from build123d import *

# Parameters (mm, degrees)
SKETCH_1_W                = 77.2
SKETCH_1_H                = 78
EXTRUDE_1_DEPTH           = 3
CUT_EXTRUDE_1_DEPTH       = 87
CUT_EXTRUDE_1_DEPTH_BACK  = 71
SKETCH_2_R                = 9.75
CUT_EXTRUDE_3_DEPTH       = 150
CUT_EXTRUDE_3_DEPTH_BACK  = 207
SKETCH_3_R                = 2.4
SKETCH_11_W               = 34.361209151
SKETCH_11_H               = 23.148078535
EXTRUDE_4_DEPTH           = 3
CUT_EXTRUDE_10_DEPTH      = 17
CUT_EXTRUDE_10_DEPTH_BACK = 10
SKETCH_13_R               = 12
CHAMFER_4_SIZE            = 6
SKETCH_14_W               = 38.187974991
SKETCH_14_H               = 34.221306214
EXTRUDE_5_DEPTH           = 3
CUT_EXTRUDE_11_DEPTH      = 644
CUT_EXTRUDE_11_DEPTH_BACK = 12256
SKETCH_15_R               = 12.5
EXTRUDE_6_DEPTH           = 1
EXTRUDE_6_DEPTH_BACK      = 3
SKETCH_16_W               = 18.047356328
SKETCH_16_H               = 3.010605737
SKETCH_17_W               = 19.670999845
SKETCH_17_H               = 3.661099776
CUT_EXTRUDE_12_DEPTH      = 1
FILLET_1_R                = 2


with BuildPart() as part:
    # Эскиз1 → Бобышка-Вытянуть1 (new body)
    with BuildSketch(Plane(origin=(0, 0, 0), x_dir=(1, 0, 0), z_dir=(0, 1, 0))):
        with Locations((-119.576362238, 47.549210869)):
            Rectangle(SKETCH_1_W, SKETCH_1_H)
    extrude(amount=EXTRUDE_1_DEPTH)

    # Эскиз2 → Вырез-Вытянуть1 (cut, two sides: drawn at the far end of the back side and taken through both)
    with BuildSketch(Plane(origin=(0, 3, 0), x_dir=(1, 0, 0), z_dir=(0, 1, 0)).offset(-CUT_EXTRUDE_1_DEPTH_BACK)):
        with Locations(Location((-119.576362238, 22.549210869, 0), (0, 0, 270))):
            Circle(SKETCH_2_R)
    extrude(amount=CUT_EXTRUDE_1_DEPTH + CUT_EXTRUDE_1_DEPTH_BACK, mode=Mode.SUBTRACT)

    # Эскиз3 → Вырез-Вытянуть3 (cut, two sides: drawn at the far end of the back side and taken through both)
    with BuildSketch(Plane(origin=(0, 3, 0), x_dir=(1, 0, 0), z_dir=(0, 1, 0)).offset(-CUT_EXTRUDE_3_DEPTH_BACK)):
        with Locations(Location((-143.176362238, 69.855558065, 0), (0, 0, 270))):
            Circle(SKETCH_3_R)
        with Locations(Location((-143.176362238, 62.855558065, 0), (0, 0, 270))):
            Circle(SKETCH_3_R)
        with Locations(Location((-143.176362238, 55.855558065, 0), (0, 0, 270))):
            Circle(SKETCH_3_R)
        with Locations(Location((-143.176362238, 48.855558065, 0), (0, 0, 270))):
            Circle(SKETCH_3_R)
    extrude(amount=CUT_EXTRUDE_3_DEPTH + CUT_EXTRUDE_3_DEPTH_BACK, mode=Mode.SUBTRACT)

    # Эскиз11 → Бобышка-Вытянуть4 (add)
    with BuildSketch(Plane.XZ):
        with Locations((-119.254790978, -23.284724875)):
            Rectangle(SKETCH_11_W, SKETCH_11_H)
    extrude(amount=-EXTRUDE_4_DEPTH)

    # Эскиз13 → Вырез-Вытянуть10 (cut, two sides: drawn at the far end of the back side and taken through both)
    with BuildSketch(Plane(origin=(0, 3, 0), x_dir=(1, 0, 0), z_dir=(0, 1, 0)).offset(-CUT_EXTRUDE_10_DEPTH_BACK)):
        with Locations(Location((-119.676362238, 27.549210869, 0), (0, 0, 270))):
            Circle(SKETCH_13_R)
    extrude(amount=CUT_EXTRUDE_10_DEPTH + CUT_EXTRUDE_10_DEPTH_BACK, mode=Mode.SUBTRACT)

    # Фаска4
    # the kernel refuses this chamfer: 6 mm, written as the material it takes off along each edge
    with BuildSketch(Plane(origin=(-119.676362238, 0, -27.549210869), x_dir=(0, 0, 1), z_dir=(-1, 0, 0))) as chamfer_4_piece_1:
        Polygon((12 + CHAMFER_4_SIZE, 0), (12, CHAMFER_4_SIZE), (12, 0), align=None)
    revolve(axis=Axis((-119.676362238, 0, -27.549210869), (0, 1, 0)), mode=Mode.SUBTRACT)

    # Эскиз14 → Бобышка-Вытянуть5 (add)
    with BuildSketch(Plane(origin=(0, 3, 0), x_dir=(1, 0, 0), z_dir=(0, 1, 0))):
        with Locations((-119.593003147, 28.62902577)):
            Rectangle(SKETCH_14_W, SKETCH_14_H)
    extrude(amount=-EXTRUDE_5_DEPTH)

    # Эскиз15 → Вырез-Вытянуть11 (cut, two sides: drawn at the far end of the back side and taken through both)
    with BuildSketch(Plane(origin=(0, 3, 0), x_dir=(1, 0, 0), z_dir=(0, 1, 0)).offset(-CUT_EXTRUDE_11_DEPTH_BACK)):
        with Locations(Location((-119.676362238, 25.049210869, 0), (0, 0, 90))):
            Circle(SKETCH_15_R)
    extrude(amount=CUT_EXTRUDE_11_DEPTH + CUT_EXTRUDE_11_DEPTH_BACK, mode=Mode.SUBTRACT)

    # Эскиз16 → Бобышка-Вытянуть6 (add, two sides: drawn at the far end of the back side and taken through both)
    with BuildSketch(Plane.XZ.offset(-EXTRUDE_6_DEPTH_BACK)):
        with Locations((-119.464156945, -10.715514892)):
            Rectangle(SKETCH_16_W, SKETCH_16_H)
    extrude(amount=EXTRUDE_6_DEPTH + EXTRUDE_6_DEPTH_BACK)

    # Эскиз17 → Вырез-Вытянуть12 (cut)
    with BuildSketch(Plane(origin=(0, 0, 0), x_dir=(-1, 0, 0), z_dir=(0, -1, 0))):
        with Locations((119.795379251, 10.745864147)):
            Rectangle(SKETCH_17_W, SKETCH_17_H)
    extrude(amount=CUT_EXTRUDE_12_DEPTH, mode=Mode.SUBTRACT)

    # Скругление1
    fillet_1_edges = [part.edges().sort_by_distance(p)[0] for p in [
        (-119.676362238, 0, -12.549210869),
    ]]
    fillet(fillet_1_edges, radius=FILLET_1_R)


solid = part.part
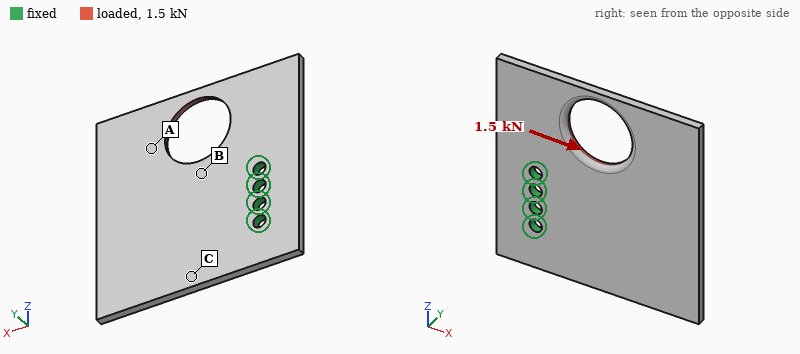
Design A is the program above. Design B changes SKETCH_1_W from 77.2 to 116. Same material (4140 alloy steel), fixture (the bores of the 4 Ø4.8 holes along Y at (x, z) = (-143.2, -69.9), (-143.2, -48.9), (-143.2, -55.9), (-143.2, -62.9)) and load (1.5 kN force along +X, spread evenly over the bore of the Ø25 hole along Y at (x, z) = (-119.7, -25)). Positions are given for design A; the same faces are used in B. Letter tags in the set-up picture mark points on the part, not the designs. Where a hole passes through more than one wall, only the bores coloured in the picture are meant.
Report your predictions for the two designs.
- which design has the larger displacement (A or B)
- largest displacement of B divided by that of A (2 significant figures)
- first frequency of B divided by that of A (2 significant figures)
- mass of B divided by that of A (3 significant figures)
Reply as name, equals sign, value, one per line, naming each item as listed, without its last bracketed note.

which design has the larger displacement = B
largest displacement of B divided by that of A = 1.2
first frequency of B divided by that of A = 0.59
mass of B divided by that of A = 1.56
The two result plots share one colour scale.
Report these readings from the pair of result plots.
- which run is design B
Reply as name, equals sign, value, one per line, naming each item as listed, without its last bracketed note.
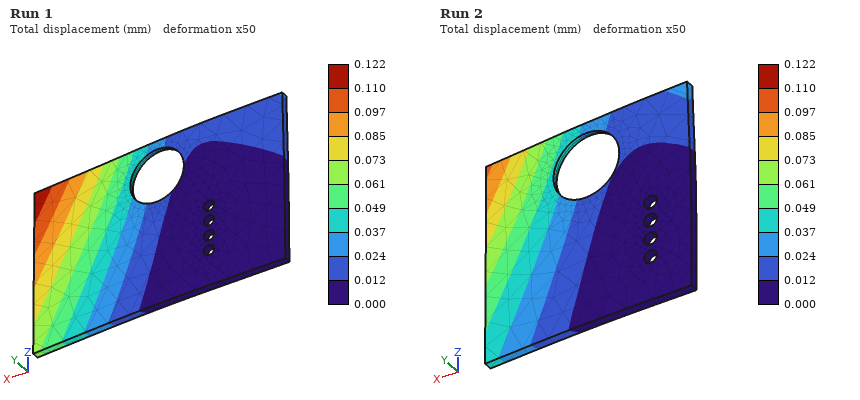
which run is design B = Run 1
